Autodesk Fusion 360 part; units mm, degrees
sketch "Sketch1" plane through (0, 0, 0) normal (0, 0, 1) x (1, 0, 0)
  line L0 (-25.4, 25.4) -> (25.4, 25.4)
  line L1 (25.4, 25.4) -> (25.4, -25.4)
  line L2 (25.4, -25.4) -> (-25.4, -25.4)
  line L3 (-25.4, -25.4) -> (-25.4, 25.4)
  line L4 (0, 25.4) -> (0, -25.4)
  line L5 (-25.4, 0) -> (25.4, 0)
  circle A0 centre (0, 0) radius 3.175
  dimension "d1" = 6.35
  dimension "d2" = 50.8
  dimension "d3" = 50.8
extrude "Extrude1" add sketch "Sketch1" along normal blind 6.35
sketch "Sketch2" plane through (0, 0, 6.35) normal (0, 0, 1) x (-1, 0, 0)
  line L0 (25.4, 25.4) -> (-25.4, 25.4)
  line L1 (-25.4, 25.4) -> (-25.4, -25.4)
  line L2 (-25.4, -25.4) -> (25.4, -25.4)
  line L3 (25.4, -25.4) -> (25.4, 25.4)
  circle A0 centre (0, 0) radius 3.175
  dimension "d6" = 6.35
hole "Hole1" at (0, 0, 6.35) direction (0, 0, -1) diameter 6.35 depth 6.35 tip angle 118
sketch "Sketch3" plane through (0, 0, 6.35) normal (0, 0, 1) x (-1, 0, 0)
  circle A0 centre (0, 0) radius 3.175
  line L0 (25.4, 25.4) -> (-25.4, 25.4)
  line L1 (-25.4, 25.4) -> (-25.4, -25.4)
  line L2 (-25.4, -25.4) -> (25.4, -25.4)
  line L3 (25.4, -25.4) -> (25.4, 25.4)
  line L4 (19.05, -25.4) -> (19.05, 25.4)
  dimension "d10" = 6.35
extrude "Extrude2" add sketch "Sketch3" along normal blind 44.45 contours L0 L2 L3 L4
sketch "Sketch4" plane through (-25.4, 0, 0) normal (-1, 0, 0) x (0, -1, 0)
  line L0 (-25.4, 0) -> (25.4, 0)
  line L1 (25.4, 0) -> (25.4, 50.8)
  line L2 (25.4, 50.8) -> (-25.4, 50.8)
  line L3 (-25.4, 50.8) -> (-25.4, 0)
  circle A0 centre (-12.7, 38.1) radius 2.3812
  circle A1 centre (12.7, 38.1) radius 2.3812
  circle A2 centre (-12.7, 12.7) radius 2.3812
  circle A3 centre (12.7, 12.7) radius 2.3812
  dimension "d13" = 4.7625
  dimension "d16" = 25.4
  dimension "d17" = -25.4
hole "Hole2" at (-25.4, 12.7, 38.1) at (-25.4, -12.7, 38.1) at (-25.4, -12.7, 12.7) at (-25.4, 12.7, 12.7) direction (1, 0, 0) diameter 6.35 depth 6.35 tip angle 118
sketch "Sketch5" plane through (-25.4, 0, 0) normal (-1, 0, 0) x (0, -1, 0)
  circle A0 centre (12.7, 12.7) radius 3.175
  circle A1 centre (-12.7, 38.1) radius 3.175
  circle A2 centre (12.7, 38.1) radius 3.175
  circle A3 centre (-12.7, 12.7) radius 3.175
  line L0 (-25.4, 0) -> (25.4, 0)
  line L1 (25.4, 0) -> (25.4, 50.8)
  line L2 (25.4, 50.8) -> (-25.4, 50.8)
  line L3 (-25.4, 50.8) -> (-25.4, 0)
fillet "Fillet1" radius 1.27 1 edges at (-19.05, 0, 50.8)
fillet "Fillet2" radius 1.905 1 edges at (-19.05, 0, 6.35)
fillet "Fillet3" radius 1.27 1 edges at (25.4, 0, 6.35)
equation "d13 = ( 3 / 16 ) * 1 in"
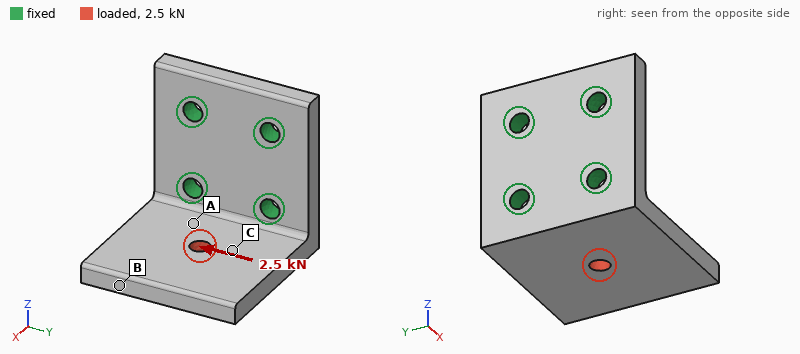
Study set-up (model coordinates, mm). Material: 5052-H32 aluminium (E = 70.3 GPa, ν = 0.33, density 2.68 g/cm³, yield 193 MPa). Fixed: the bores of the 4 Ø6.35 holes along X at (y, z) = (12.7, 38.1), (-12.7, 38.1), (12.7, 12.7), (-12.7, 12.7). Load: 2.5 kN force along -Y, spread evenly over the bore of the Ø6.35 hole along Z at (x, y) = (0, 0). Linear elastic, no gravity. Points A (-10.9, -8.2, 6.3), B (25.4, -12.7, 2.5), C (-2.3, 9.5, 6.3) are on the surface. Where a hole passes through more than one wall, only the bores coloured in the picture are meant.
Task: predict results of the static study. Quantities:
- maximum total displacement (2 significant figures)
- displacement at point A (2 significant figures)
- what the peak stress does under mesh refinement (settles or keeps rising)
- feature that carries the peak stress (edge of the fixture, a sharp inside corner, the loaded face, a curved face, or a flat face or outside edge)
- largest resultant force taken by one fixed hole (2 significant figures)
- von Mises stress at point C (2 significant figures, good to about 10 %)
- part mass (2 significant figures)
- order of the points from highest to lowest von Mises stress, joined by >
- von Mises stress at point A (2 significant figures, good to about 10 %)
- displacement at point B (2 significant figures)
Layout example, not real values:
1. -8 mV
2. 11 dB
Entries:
1. 61 µm
2. 17 µm
3. keeps rising
4. edge of the fixture
5. 2.3 kN
6. 21 MPa
7. 80 g
8. A > C > B
9. 30 MPa
10. 52 µm
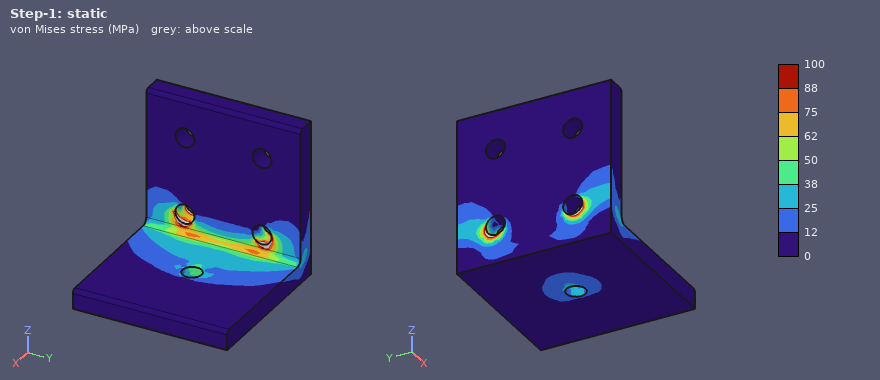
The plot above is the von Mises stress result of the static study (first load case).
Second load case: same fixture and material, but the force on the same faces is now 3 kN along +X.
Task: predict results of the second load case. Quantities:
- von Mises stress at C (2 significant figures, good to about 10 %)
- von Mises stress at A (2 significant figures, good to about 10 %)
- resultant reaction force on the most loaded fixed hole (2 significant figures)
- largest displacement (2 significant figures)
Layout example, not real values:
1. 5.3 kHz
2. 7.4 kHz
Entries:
1. 8.8 MPa
2. 14 MPa
3. 1.6 kN
4. 81 µm
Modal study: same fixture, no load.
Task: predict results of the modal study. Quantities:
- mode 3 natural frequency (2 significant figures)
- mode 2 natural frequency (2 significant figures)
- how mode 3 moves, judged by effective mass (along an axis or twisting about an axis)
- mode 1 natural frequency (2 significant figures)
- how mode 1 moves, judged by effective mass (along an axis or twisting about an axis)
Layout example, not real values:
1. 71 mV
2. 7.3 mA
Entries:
1. 6400 Hz
2. 4500 Hz
3. along Y
4. 1900 Hz
5. along Z
